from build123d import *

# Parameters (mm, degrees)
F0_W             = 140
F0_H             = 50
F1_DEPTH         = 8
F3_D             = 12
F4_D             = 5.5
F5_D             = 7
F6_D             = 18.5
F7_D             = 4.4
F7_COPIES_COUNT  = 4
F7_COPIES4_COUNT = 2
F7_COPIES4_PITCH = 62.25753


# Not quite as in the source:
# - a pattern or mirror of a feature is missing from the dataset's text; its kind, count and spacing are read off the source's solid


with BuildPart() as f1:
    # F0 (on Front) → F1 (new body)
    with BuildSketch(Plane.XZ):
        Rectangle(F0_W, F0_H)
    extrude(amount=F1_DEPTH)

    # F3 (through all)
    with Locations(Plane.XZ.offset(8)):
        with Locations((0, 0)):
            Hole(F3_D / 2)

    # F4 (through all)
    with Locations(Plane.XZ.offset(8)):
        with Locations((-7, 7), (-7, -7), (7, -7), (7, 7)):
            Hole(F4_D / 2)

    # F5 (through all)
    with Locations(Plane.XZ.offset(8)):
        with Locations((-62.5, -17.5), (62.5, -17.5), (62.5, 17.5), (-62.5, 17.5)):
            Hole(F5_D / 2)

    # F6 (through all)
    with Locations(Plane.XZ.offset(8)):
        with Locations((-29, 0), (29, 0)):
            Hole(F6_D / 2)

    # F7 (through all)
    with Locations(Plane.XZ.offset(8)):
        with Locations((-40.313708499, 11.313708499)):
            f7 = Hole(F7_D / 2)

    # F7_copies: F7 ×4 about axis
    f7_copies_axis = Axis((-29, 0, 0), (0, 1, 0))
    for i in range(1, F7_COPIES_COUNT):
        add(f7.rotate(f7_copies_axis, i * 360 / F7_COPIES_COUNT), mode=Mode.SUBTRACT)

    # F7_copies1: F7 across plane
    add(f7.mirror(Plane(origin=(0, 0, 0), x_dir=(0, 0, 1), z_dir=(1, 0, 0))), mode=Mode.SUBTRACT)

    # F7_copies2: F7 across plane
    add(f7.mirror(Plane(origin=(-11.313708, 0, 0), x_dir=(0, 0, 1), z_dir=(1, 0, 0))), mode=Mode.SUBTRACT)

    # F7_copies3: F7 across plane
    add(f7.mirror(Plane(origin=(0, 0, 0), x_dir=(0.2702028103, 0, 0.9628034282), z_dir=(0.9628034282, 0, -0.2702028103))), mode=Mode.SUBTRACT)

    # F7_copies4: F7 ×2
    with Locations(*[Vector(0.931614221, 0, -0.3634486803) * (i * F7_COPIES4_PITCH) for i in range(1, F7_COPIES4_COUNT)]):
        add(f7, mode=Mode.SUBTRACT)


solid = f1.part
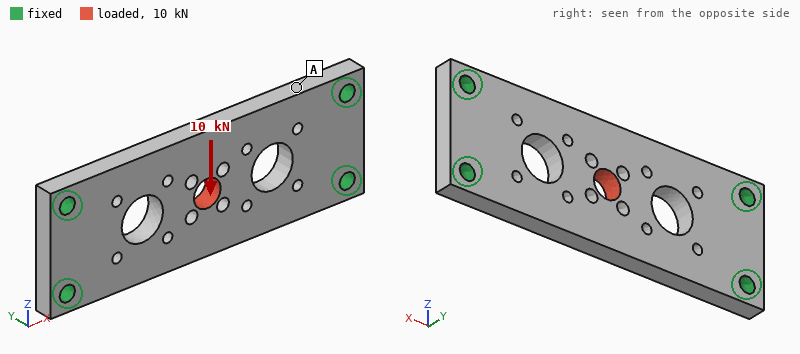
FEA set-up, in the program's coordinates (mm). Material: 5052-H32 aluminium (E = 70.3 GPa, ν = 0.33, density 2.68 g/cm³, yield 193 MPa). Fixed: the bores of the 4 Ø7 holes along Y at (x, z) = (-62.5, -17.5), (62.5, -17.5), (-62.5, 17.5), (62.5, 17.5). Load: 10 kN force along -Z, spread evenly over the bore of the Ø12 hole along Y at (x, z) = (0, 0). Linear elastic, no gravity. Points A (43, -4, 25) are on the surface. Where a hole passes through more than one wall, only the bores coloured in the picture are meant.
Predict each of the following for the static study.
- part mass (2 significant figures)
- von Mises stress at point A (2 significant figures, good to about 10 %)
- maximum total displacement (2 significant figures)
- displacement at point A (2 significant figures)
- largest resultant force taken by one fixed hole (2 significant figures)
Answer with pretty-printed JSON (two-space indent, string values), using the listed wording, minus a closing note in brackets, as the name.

{
  "part mass": "130 g",
  "von Mises stress at point A": "39 MPa",
  "maximum total displacement": "80 µm",
  "displacement at point A": "22 µm",
  "largest resultant force taken by one fixed hole": "4.7 kN"
}
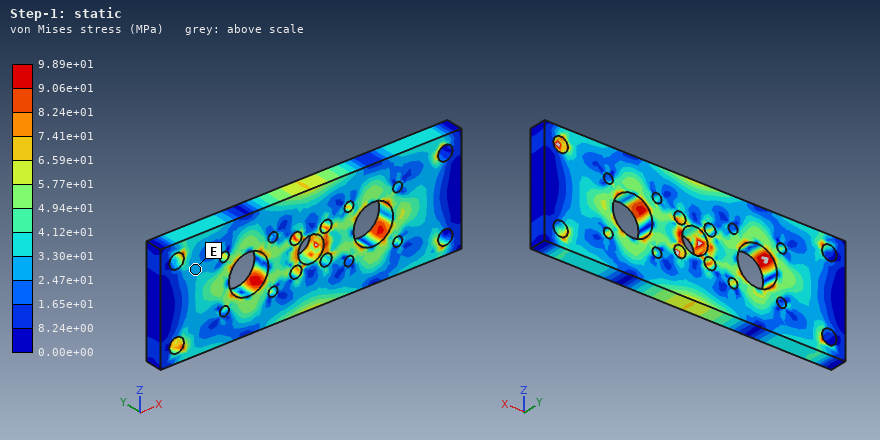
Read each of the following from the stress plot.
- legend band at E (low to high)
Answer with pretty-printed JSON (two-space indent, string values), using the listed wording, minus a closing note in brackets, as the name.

{
  "legend band at E": "2.47e+01 to 3.30e+01 MPa"
}
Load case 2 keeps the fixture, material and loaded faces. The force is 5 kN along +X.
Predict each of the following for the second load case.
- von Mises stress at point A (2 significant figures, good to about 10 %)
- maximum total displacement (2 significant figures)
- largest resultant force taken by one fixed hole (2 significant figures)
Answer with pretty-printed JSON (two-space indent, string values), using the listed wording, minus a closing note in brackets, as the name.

{
  "von Mises stress at point A": "10 MPa",
  "maximum total displacement": "15 µm",
  "largest resultant force taken by one fixed hole": "1.3 kN"
}
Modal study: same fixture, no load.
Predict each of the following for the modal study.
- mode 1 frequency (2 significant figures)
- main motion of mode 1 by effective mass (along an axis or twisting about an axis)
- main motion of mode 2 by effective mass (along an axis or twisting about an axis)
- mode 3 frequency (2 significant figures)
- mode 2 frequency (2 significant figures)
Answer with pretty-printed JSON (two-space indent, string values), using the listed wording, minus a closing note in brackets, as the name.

{
  "mode 1 frequency": "2700 Hz",
  "main motion of mode 1 by effective mass": "along Y",
  "main motion of mode 2 by effective mass": "twisting about X",
  "mode 3 frequency": "7100 Hz",
  "mode 2 frequency": "4500 Hz"
}
